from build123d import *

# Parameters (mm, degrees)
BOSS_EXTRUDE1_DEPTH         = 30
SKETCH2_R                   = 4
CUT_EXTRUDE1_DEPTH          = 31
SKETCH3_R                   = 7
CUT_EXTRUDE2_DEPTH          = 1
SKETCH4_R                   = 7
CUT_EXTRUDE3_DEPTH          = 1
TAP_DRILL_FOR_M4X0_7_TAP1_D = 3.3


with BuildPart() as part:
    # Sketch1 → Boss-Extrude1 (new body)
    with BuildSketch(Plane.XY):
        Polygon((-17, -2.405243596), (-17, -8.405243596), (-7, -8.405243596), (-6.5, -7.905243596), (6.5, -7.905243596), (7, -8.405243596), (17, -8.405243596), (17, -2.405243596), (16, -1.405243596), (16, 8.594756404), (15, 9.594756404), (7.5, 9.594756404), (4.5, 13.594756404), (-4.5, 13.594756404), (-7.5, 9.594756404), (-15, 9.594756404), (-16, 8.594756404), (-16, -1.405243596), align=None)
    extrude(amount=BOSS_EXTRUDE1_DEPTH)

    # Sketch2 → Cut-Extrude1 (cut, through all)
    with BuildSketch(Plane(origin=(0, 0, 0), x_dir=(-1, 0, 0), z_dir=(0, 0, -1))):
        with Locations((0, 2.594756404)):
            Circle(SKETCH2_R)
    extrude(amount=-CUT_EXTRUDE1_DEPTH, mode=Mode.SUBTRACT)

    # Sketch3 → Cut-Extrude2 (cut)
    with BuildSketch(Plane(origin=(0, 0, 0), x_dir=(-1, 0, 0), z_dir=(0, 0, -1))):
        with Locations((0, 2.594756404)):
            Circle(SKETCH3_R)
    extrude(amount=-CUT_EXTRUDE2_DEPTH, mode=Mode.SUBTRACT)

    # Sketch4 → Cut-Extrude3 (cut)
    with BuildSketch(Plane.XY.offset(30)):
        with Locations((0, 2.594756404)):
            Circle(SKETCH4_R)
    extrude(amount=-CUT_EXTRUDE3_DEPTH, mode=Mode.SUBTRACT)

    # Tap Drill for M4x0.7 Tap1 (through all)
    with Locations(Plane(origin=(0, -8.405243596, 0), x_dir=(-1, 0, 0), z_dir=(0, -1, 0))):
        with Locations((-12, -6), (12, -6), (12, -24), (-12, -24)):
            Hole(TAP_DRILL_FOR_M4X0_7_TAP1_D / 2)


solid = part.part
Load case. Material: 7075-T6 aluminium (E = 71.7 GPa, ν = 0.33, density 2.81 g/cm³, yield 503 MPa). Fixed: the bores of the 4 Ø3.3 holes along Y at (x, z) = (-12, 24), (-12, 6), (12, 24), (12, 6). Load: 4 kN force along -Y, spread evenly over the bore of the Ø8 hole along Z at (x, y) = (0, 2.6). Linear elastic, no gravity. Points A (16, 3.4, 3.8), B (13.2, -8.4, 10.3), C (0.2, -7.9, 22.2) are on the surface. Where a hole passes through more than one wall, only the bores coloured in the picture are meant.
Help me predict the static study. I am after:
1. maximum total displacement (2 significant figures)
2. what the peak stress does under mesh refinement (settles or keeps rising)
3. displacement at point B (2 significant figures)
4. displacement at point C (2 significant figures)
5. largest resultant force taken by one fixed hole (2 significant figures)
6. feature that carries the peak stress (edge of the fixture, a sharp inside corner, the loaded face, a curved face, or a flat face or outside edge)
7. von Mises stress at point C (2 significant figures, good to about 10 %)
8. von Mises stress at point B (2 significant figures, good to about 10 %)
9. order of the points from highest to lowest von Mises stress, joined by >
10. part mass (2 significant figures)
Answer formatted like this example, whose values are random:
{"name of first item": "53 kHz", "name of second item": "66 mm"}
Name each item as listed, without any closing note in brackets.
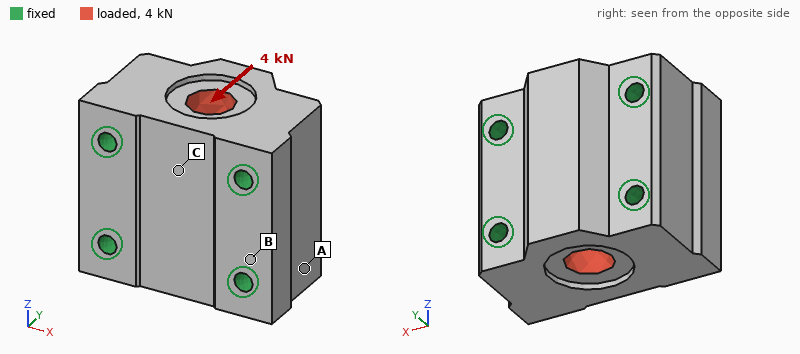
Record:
{"maximum total displacement": "2.1 µm", "what the peak stress does under mesh refinement": "keeps rising", "displacement at point B": "0.47 µm", "displacement at point C": "1.6 µm", "largest resultant force taken by one fixed hole": "1.0 kN", "feature that carries the peak stress": "edge of the fixture", "von Mises stress at point C": "6.7 MPa", "von Mises stress at point B": "4.0 MPa", "order of the points from highest to lowest von Mises stress, joined by >": "C > B > A", "part mass": "46 g"}
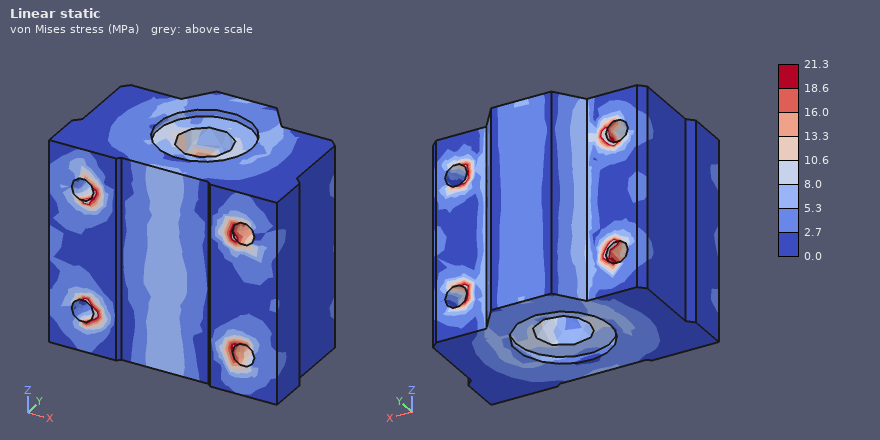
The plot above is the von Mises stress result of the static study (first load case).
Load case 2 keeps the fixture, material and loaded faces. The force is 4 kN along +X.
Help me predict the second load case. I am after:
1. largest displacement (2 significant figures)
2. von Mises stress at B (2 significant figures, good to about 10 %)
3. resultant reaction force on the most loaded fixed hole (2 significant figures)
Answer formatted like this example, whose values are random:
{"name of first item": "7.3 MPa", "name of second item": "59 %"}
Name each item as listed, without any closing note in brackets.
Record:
{"largest displacement": "1.1 µm", "von Mises stress at B": "2.5 MPa", "resultant reaction force on the most loaded fixed hole": "1.0 kN"}
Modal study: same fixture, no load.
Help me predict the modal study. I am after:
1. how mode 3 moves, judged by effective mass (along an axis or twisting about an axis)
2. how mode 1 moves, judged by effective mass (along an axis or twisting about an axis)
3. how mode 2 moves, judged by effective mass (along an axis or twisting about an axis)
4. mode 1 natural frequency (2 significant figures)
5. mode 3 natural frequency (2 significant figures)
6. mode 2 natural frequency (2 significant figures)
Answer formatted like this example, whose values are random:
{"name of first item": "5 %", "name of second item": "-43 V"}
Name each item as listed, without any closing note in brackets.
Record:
{"how mode 3 moves, judged by effective mass": "along Z", "how mode 1 moves, judged by effective mass": "along Z", "how mode 2 moves, judged by effective mass": "along Y", "mode 1 natural frequency": "50 kHz", "mode 3 natural frequency": "62 kHz", "mode 2 natural frequency": "54 kHz"}
